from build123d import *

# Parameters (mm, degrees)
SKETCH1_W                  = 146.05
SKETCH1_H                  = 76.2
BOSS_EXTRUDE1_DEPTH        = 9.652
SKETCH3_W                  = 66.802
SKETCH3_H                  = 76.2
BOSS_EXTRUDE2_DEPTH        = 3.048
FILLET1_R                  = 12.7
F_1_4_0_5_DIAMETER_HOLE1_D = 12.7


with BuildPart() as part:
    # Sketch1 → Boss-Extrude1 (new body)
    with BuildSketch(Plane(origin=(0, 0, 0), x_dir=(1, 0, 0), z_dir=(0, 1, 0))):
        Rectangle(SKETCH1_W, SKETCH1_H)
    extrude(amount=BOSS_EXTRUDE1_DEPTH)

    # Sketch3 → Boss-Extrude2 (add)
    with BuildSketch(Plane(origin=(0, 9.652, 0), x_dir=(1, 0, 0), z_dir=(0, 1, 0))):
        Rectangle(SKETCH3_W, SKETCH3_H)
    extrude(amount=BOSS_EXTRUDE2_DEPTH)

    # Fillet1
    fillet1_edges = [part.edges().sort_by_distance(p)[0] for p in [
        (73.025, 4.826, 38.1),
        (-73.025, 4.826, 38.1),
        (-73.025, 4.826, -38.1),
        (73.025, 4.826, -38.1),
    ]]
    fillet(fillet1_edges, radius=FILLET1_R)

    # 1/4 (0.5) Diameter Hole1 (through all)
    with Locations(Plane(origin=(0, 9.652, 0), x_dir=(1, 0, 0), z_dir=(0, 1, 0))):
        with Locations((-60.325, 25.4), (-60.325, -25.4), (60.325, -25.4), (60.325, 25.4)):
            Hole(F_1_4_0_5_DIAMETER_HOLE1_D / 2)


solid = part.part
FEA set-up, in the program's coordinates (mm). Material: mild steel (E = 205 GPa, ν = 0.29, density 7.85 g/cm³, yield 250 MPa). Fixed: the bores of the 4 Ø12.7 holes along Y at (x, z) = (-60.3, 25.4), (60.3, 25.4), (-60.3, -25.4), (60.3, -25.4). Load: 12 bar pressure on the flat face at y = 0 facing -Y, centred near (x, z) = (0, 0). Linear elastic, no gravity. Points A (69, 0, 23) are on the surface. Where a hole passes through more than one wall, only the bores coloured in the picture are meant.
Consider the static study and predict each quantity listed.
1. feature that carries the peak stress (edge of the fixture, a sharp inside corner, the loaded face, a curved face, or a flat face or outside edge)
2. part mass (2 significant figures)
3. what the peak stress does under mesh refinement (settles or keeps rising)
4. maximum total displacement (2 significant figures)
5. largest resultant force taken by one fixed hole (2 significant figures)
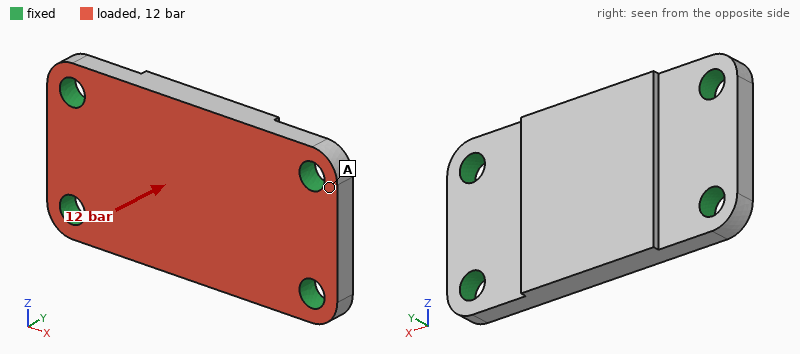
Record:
edge of the fixture
920 g
keeps rising
27 µm
3.3 kN
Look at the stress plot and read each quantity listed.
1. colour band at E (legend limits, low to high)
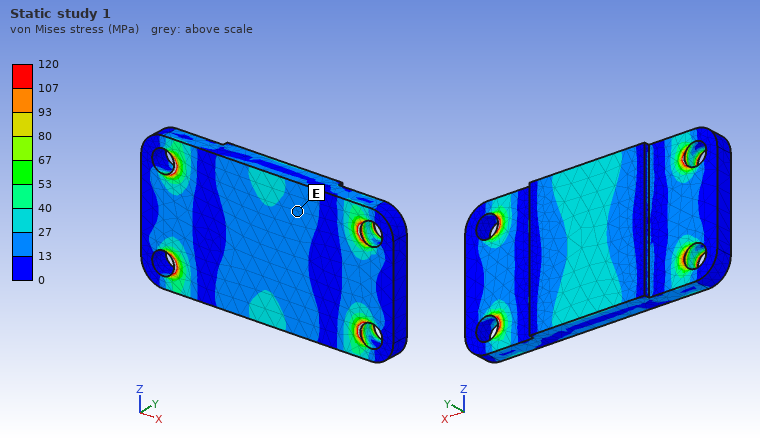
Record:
13 to 27 MPa
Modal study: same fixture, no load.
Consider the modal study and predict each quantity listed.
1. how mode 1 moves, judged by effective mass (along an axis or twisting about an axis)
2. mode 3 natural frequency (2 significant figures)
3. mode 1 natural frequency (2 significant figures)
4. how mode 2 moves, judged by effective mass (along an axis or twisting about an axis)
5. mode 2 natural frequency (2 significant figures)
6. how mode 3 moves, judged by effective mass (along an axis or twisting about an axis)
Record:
along Y
10 kHz
3900 Hz
twisting about X
5400 Hz
twisting about Z
